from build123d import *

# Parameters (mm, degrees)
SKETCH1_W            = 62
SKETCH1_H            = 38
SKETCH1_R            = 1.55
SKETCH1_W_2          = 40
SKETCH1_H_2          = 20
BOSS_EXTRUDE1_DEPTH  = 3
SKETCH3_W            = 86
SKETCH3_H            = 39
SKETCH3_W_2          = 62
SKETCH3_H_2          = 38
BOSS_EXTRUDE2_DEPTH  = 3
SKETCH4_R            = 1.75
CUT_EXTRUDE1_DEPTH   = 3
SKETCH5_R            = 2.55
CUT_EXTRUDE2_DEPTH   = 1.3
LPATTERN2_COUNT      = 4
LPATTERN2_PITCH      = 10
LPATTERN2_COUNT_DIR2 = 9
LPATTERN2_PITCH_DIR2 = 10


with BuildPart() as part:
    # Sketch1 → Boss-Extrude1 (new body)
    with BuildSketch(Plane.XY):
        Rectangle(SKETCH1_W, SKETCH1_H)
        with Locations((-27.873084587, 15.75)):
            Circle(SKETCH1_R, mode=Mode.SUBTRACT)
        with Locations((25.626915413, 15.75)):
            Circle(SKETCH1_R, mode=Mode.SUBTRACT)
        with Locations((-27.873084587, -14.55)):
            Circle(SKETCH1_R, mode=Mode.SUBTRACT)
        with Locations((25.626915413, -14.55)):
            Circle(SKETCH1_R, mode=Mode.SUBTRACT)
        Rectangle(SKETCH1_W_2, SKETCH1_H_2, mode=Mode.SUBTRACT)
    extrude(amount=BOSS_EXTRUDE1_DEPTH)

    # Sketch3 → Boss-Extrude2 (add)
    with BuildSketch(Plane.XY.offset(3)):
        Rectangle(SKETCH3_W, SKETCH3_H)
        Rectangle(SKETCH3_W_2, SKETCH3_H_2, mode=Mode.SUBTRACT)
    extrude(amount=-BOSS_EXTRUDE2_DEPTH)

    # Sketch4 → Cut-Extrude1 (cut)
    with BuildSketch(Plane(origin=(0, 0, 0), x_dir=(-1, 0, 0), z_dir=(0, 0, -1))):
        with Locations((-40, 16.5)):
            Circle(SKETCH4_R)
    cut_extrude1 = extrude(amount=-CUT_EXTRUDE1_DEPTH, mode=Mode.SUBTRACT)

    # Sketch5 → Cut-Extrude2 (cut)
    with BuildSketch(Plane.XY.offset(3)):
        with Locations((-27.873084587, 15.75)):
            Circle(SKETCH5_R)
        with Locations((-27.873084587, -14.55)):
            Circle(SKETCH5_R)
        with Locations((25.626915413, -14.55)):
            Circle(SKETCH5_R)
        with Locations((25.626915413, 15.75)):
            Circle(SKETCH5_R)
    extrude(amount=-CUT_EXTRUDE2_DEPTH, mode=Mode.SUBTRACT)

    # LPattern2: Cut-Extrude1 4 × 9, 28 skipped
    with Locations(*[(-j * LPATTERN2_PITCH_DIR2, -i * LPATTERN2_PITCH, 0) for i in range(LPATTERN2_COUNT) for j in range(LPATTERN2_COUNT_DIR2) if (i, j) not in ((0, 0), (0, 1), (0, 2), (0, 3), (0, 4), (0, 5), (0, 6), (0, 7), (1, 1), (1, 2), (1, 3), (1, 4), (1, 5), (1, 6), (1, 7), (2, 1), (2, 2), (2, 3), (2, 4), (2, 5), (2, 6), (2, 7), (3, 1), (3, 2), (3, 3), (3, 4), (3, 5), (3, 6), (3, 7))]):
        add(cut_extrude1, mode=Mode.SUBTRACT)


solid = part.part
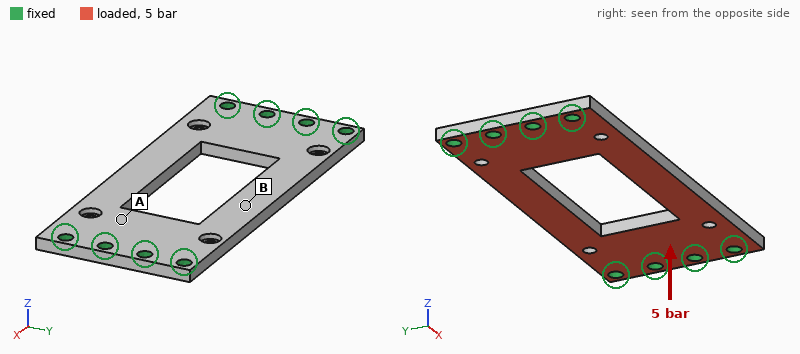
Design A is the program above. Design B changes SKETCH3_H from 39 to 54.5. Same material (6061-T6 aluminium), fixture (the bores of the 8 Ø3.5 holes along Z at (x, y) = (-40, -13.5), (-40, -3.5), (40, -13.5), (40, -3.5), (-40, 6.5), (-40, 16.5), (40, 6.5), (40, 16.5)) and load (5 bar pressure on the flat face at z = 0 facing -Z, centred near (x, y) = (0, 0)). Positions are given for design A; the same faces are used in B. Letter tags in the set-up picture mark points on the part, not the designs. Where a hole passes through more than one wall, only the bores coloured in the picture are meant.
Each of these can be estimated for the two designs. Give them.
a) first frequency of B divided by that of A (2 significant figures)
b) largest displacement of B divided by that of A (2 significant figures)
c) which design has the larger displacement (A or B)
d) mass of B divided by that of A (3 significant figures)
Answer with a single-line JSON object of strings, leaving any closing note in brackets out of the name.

{"first frequency of B divided by that of A": "0.87", "largest displacement of B divided by that of A": "1.4", "which design has the larger displacement": "B", "mass of B divided by that of A": "1.55"}
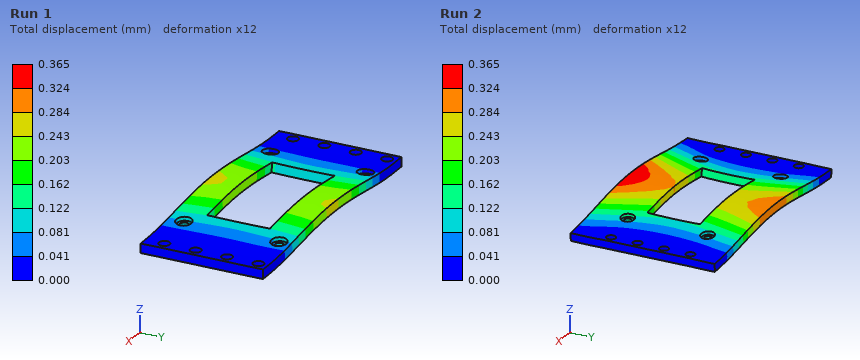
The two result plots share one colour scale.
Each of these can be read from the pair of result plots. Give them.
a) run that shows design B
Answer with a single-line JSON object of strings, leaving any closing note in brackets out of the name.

{"run that shows design B": "Run 2"}
